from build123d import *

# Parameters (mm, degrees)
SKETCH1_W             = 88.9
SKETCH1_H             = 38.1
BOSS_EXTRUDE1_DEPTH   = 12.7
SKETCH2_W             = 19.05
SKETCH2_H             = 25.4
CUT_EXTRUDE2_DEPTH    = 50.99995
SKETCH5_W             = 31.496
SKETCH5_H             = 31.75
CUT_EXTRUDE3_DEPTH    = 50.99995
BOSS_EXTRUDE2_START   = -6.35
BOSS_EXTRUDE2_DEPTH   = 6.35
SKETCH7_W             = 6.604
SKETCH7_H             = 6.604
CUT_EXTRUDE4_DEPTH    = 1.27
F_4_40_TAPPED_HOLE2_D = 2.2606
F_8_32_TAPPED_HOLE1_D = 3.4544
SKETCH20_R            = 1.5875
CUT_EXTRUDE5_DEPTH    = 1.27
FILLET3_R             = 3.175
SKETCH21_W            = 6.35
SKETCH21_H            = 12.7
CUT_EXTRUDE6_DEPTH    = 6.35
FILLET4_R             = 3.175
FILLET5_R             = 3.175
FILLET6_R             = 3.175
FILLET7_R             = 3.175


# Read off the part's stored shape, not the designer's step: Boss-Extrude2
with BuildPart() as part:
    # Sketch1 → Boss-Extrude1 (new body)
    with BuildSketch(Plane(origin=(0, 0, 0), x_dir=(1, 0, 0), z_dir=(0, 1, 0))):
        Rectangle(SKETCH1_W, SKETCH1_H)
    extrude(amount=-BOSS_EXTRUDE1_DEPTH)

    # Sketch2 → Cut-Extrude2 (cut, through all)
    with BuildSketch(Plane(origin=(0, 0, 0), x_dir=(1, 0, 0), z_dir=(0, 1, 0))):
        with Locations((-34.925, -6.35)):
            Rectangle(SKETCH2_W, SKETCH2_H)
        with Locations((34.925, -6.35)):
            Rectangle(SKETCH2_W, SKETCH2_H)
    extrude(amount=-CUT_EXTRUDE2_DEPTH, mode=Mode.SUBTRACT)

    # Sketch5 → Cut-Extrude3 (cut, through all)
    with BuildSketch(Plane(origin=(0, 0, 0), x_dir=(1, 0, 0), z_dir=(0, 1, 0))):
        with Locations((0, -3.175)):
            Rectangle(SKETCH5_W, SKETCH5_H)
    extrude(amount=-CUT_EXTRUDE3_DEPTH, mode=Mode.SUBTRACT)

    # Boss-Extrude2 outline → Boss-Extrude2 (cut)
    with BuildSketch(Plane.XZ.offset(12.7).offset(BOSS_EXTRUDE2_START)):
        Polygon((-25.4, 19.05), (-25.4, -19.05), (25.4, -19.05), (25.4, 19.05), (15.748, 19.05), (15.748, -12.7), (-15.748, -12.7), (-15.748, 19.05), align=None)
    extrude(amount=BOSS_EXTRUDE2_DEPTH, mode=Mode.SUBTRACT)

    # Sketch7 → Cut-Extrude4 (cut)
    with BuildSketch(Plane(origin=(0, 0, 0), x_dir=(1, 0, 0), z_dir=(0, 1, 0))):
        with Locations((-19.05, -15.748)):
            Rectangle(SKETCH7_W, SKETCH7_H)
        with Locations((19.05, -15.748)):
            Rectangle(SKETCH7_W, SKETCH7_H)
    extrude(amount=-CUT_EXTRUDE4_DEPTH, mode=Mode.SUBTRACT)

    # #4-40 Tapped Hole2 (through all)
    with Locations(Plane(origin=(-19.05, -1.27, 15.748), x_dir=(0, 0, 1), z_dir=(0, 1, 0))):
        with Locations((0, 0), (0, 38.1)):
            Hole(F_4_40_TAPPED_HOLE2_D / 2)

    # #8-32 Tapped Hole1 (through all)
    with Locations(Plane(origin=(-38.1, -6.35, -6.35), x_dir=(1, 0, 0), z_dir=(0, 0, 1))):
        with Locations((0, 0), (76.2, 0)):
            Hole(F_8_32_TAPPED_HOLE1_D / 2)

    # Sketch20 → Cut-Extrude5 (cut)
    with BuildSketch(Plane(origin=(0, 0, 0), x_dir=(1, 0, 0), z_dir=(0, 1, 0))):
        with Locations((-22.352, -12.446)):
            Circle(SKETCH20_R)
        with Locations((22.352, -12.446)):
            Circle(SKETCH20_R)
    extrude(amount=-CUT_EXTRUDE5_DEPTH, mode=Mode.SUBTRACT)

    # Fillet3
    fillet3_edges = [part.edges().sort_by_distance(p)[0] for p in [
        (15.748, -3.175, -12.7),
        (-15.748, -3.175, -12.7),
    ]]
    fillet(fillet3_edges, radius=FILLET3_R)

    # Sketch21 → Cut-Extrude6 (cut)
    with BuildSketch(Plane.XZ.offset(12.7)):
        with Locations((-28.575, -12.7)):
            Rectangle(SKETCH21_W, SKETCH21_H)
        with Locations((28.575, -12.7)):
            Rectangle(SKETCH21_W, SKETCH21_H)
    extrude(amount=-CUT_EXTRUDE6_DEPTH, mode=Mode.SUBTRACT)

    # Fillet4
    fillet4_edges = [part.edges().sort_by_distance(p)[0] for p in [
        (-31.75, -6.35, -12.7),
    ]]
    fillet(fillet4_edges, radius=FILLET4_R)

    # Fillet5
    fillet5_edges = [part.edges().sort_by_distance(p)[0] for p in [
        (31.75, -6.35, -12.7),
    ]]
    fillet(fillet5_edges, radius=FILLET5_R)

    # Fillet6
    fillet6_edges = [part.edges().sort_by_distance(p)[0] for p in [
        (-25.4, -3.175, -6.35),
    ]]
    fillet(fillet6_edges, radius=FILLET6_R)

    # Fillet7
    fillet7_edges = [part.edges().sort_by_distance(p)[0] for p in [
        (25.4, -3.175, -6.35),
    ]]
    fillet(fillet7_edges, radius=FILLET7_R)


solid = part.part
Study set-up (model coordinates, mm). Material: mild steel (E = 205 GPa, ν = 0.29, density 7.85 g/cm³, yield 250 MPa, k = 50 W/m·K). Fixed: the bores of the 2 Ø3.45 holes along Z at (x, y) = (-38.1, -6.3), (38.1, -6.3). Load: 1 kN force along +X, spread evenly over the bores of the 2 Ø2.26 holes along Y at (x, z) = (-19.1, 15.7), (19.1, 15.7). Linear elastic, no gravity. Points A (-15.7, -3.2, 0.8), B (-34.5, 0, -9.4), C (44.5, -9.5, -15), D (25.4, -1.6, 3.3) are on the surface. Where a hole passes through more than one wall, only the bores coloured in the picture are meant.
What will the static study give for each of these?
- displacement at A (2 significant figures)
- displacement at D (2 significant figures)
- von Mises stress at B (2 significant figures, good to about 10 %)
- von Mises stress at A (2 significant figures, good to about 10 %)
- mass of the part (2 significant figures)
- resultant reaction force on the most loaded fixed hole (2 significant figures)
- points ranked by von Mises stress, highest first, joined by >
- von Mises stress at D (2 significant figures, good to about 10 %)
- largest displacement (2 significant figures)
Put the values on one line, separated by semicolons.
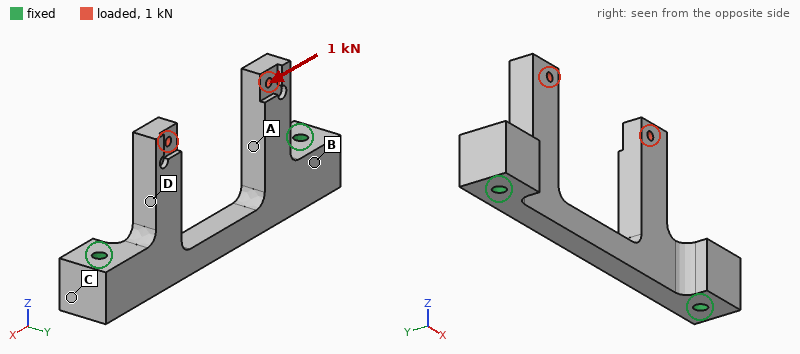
18 µm; 17 µm; 24 MPa; 77 MPa; 85 g; 540 N; A > D > B > C; 62 MPa; 52 µm
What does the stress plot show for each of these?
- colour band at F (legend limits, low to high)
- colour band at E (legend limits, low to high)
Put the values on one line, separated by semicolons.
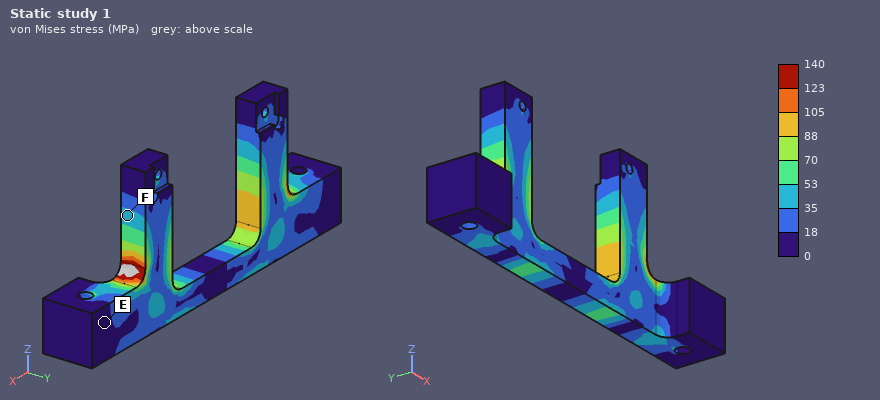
35 to 53 MPa; 0 to 18 MPa
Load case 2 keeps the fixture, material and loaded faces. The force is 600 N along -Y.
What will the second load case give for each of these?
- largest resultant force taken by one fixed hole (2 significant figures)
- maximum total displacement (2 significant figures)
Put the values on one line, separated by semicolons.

310 N; 0.10 mm
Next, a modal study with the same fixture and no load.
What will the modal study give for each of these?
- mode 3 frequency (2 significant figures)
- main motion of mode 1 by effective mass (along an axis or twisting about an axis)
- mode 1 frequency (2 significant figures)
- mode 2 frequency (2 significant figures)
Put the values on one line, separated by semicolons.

6400 Hz; along Y; 4200 Hz; 4400 Hz
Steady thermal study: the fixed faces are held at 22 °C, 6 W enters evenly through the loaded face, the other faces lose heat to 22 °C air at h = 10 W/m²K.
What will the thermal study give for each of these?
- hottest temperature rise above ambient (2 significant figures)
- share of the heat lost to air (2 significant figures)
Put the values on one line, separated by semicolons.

35 K; 9.5 %
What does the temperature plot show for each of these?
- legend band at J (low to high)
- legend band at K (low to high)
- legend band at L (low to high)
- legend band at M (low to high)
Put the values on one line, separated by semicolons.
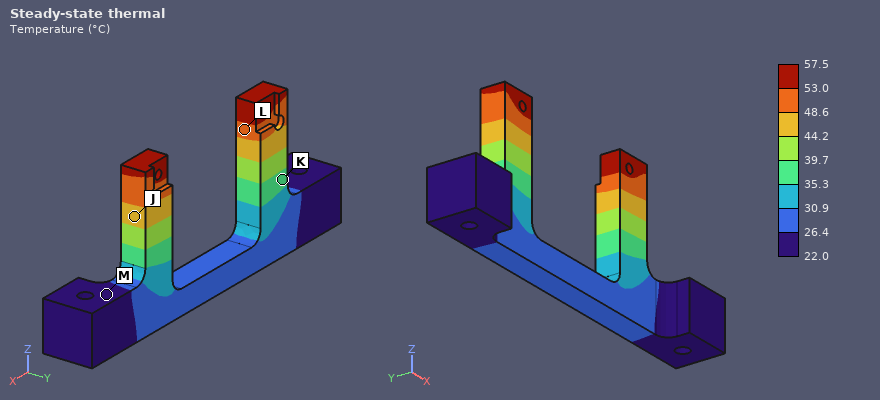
44.2 to 48.6 °C; 35.3 to 39.7 °C; 48.6 to 53.0 °C; 22.0 to 26.4 °C
